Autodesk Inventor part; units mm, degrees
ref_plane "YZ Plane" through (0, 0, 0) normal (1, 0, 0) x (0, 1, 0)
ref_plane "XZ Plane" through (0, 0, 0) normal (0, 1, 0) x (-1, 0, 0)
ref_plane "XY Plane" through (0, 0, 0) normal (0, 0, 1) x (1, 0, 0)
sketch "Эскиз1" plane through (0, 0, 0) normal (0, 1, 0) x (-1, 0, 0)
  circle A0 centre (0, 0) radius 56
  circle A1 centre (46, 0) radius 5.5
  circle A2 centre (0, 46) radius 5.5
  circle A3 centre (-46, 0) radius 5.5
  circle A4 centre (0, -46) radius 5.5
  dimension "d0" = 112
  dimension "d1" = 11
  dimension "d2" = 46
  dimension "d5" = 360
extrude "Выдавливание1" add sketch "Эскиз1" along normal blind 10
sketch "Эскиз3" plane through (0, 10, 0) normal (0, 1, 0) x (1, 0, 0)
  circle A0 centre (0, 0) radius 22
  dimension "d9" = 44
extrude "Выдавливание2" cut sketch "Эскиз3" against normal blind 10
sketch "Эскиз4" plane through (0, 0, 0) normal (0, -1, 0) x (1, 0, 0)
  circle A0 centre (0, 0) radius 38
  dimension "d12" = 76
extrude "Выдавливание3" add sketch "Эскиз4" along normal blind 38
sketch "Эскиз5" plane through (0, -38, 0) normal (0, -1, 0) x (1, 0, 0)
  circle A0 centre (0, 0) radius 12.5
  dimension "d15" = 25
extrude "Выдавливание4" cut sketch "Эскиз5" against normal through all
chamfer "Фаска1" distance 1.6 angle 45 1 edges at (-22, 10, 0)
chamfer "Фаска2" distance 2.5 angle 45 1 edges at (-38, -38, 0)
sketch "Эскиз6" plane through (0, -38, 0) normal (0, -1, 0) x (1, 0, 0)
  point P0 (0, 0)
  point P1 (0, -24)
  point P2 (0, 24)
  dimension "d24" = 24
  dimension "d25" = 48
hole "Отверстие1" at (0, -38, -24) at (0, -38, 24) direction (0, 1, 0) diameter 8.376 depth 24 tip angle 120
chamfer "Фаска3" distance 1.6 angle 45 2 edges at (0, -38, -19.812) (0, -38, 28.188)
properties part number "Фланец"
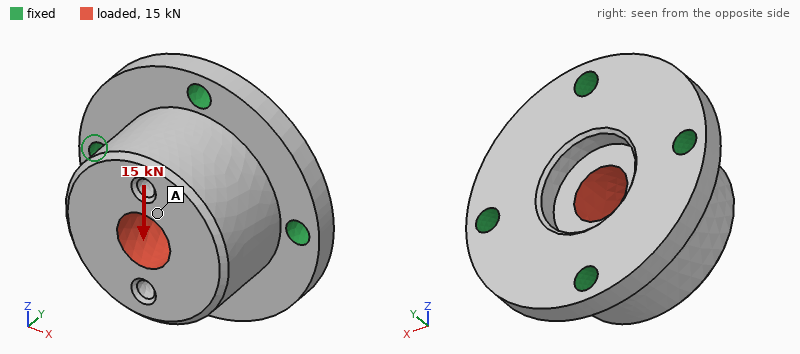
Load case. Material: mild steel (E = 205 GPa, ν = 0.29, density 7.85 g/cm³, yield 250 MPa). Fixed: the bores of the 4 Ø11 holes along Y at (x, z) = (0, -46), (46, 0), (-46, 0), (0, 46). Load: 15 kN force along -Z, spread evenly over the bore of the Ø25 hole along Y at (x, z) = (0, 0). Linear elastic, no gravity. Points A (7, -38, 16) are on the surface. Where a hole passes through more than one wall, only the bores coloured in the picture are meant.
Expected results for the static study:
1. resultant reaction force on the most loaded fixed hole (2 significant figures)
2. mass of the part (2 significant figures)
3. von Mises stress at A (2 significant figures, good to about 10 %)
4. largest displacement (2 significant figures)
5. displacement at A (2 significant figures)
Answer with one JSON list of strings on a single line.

["6.4 kN", "1.8 kg", "8.7 MPa", "6.1 µm", "5.8 µm"]
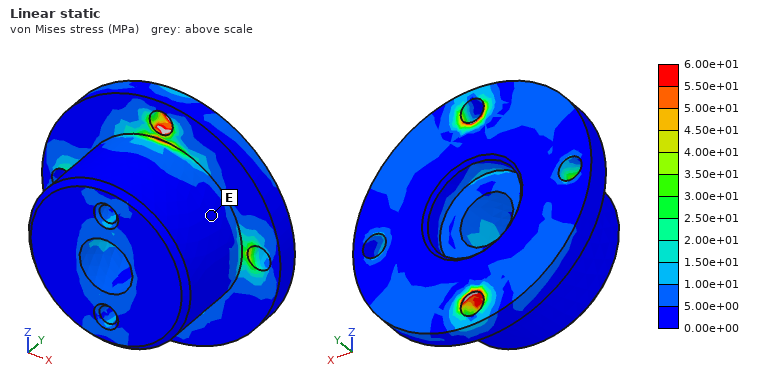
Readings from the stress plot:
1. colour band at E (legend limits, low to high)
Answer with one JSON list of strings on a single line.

["0.00e+00 to 5.00e+00 MPa"]
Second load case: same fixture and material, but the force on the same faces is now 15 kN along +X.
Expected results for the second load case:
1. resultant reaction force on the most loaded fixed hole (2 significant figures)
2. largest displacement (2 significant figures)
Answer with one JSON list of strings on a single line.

["6.4 kN", "6.1 µm"]
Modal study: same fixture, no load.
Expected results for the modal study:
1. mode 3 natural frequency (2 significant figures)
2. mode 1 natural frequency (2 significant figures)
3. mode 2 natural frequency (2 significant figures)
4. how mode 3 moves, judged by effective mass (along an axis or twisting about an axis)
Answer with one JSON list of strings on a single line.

["9100 Hz", "7800 Hz", "7800 Hz", "along Y"]
